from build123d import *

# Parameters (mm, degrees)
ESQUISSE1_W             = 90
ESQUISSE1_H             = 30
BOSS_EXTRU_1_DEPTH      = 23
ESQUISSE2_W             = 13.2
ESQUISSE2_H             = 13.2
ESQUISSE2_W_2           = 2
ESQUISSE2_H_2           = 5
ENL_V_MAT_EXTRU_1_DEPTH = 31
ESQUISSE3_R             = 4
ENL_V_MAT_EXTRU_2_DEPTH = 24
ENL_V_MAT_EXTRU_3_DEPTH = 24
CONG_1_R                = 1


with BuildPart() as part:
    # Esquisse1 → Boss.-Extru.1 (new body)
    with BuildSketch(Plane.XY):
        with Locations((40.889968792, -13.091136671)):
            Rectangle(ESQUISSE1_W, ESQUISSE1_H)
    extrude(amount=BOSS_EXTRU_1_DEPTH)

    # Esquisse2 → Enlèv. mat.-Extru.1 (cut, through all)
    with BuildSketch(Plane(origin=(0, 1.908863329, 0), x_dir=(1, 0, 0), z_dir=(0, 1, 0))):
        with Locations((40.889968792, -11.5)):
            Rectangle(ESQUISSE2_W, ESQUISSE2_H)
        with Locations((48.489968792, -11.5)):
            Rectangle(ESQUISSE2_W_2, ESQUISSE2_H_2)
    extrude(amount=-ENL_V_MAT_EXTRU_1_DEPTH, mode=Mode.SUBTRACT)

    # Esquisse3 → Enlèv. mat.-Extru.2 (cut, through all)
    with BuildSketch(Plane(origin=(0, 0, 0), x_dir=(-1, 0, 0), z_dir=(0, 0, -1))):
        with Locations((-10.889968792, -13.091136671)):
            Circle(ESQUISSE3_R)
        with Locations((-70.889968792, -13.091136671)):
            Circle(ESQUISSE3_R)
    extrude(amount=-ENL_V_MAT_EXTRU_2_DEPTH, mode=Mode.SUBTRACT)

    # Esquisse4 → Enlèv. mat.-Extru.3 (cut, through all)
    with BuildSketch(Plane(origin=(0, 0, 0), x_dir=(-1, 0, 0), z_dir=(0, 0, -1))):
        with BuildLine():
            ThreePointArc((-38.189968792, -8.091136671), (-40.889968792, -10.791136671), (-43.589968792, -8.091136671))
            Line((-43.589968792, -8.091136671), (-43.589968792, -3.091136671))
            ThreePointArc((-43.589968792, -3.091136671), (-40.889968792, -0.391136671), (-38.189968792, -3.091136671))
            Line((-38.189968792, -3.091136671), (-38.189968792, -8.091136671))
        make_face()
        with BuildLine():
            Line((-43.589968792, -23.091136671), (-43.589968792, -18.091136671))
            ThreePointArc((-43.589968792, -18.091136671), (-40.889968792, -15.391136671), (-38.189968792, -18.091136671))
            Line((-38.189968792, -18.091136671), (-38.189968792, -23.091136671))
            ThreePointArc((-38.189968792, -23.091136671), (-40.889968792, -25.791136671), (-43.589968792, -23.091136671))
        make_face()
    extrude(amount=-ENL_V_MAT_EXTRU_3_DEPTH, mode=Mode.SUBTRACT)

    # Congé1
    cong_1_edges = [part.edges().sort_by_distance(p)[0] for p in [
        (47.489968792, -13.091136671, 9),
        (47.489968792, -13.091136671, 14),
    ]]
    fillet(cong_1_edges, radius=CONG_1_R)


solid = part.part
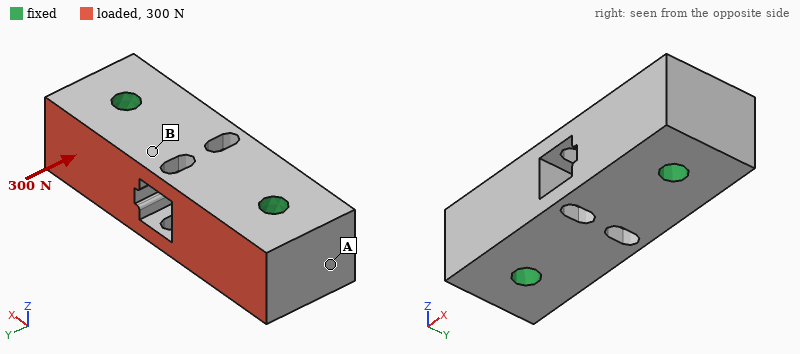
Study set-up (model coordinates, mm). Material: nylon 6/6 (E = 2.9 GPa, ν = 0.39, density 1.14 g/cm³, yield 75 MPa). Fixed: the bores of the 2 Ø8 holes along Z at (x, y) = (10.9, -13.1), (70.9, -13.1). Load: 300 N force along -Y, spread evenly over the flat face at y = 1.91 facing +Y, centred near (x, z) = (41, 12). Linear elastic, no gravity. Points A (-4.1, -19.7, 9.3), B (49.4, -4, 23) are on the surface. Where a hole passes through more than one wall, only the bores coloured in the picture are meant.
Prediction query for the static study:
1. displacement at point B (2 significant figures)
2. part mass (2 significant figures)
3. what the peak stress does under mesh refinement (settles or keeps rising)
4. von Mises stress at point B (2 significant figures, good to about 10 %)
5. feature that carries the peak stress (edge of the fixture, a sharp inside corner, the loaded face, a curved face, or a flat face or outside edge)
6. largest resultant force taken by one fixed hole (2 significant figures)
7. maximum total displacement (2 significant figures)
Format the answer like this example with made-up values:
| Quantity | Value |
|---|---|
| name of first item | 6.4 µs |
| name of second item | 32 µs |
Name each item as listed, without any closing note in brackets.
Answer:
| Quantity | Value |
|---|---|
| displacement at point B | 4.2 µm |
| part mass | 61 g |
| what the peak stress does under mesh refinement | keeps rising |
| von Mises stress at point B | 0.23 MPa |
| feature that carries the peak stress | a sharp inside corner |
| largest resultant force taken by one fixed hole | 150 N |
| maximum total displacement | 5.1 µm |
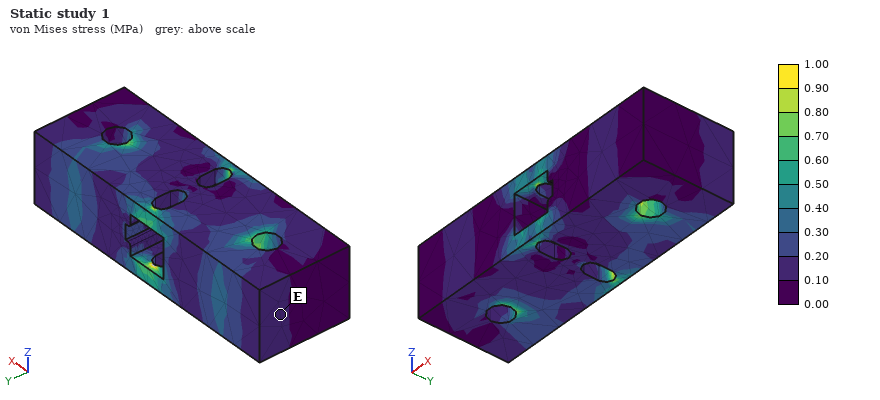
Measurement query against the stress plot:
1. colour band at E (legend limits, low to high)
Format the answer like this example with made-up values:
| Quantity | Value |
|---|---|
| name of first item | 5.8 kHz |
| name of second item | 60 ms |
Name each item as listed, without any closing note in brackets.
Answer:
| Quantity | Value |
|---|---|
| colour band at E | 0.10 to 0.20 MPa |
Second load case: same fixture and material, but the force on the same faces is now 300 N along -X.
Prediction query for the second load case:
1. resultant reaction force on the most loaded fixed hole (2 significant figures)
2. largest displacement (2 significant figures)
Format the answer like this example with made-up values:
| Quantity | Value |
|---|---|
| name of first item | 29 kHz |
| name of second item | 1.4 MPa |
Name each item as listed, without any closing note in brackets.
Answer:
| Quantity | Value |
|---|---|
| resultant reaction force on the most loaded fixed hole | 160 N |
| largest displacement | 6.9 µm |
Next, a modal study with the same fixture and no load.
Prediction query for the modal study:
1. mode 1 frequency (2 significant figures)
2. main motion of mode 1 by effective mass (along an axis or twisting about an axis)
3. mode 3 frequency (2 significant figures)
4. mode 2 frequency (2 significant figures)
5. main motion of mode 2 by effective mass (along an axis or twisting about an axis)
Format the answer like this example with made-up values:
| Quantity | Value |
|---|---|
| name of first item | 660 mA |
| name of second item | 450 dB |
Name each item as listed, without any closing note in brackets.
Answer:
| Quantity | Value |
|---|---|
| mode 1 frequency | 5100 Hz |
| main motion of mode 1 by effective mass | along Y |
| mode 3 frequency | 7400 Hz |
| mode 2 frequency | 6600 Hz |
| main motion of mode 2 by effective mass | along Z |
